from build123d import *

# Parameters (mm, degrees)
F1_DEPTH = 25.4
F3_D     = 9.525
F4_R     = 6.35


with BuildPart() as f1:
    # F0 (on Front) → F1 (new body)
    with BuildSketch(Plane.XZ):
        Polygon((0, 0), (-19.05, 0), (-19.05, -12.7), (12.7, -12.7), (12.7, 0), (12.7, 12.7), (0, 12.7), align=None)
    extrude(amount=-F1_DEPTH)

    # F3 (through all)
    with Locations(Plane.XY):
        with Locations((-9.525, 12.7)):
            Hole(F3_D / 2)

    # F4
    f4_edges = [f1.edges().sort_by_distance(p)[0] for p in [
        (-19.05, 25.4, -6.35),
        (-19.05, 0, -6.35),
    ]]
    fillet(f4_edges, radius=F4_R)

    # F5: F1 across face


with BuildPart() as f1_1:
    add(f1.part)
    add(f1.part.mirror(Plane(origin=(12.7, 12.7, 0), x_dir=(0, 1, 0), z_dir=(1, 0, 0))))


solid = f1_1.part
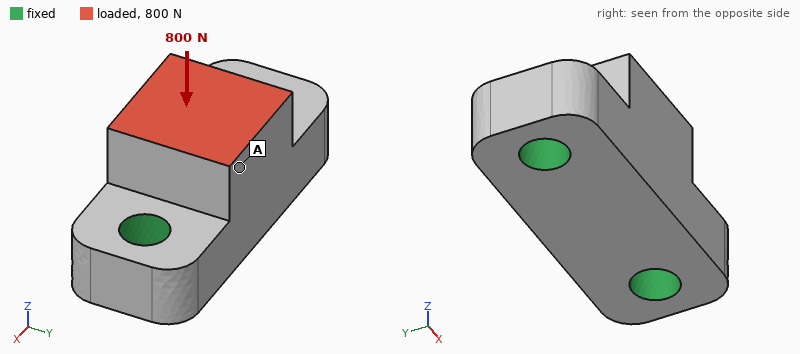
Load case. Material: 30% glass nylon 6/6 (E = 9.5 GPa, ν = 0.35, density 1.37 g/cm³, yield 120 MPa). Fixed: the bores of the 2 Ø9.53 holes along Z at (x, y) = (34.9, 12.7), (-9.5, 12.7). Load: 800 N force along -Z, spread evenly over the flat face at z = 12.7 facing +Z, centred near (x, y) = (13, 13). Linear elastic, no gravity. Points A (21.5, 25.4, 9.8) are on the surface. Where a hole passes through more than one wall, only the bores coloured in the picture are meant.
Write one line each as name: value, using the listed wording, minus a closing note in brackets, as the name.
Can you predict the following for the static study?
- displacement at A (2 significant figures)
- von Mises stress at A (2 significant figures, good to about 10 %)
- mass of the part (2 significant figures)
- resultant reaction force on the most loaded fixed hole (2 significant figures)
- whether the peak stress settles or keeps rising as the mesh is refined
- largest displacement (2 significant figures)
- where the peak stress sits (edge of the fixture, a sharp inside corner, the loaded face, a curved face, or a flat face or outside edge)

displacement at A: 7.4 µm
von Mises stress at A: 1.3 MPa
mass of the part: 36 g
resultant reaction force on the most loaded fixed hole: 420 N
whether the peak stress settles or keeps rising as the mesh is refined: keeps rising
largest displacement: 8.0 µm
where the peak stress sits: edge of the fixture
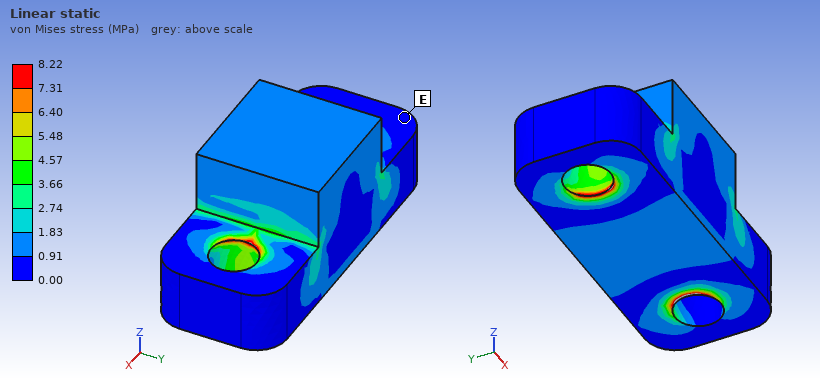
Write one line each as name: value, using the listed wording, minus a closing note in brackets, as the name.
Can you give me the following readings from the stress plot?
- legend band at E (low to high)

legend band at E: 0.00 to 0.91 MPa
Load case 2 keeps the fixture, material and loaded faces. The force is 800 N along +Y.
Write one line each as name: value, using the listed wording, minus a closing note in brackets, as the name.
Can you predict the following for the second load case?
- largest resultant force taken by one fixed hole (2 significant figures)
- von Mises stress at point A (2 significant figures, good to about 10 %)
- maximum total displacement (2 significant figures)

largest resultant force taken by one fixed hole: 400 N
von Mises stress at point A: 1.7 MPa
maximum total displacement: 54 µm
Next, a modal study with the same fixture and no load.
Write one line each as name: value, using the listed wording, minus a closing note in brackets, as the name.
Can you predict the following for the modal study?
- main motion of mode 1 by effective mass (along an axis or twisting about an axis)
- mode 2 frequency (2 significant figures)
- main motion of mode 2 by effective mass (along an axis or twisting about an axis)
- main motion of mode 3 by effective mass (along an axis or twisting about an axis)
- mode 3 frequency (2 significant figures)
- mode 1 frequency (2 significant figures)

main motion of mode 1 by effective mass: along Y
mode 2 frequency: 12 kHz
main motion of mode 2 by effective mass: along Z
main motion of mode 3 by effective mass: along X
mode 3 frequency: 14 kHz
mode 1 frequency: 7300 Hz
